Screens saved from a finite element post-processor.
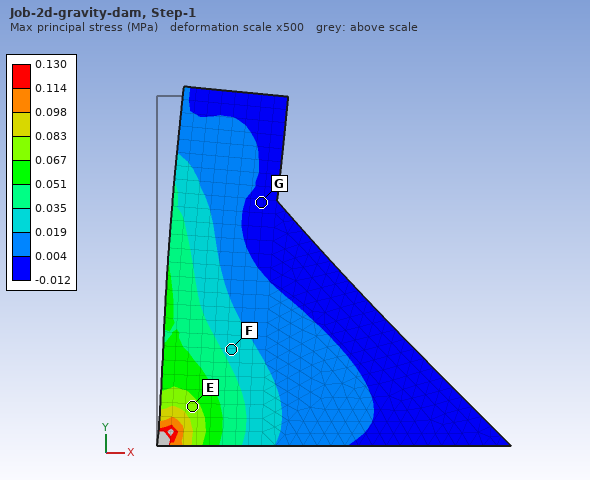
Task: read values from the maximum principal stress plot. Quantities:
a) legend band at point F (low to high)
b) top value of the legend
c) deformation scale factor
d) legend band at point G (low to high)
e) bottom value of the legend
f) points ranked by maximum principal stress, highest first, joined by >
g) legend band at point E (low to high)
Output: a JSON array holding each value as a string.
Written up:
["0.019 to 0.035 MPa", "0.130 MPa", "500", "-0.012 to 0.004 MPa", "-0.012 MPa", "E > F > G", "0.067 to 0.083 MPa"]
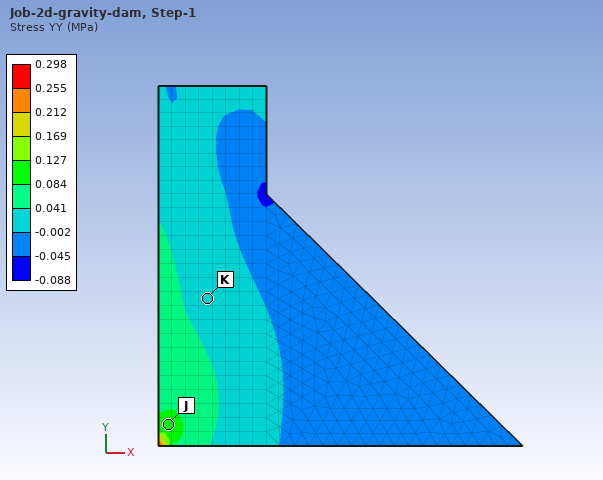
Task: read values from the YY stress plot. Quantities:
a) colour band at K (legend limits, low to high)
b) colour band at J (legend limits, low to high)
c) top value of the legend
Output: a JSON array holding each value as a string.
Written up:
["-0.002 to 0.041 MPa", "0.084 to 0.127 MPa", "0.298 MPa"]
